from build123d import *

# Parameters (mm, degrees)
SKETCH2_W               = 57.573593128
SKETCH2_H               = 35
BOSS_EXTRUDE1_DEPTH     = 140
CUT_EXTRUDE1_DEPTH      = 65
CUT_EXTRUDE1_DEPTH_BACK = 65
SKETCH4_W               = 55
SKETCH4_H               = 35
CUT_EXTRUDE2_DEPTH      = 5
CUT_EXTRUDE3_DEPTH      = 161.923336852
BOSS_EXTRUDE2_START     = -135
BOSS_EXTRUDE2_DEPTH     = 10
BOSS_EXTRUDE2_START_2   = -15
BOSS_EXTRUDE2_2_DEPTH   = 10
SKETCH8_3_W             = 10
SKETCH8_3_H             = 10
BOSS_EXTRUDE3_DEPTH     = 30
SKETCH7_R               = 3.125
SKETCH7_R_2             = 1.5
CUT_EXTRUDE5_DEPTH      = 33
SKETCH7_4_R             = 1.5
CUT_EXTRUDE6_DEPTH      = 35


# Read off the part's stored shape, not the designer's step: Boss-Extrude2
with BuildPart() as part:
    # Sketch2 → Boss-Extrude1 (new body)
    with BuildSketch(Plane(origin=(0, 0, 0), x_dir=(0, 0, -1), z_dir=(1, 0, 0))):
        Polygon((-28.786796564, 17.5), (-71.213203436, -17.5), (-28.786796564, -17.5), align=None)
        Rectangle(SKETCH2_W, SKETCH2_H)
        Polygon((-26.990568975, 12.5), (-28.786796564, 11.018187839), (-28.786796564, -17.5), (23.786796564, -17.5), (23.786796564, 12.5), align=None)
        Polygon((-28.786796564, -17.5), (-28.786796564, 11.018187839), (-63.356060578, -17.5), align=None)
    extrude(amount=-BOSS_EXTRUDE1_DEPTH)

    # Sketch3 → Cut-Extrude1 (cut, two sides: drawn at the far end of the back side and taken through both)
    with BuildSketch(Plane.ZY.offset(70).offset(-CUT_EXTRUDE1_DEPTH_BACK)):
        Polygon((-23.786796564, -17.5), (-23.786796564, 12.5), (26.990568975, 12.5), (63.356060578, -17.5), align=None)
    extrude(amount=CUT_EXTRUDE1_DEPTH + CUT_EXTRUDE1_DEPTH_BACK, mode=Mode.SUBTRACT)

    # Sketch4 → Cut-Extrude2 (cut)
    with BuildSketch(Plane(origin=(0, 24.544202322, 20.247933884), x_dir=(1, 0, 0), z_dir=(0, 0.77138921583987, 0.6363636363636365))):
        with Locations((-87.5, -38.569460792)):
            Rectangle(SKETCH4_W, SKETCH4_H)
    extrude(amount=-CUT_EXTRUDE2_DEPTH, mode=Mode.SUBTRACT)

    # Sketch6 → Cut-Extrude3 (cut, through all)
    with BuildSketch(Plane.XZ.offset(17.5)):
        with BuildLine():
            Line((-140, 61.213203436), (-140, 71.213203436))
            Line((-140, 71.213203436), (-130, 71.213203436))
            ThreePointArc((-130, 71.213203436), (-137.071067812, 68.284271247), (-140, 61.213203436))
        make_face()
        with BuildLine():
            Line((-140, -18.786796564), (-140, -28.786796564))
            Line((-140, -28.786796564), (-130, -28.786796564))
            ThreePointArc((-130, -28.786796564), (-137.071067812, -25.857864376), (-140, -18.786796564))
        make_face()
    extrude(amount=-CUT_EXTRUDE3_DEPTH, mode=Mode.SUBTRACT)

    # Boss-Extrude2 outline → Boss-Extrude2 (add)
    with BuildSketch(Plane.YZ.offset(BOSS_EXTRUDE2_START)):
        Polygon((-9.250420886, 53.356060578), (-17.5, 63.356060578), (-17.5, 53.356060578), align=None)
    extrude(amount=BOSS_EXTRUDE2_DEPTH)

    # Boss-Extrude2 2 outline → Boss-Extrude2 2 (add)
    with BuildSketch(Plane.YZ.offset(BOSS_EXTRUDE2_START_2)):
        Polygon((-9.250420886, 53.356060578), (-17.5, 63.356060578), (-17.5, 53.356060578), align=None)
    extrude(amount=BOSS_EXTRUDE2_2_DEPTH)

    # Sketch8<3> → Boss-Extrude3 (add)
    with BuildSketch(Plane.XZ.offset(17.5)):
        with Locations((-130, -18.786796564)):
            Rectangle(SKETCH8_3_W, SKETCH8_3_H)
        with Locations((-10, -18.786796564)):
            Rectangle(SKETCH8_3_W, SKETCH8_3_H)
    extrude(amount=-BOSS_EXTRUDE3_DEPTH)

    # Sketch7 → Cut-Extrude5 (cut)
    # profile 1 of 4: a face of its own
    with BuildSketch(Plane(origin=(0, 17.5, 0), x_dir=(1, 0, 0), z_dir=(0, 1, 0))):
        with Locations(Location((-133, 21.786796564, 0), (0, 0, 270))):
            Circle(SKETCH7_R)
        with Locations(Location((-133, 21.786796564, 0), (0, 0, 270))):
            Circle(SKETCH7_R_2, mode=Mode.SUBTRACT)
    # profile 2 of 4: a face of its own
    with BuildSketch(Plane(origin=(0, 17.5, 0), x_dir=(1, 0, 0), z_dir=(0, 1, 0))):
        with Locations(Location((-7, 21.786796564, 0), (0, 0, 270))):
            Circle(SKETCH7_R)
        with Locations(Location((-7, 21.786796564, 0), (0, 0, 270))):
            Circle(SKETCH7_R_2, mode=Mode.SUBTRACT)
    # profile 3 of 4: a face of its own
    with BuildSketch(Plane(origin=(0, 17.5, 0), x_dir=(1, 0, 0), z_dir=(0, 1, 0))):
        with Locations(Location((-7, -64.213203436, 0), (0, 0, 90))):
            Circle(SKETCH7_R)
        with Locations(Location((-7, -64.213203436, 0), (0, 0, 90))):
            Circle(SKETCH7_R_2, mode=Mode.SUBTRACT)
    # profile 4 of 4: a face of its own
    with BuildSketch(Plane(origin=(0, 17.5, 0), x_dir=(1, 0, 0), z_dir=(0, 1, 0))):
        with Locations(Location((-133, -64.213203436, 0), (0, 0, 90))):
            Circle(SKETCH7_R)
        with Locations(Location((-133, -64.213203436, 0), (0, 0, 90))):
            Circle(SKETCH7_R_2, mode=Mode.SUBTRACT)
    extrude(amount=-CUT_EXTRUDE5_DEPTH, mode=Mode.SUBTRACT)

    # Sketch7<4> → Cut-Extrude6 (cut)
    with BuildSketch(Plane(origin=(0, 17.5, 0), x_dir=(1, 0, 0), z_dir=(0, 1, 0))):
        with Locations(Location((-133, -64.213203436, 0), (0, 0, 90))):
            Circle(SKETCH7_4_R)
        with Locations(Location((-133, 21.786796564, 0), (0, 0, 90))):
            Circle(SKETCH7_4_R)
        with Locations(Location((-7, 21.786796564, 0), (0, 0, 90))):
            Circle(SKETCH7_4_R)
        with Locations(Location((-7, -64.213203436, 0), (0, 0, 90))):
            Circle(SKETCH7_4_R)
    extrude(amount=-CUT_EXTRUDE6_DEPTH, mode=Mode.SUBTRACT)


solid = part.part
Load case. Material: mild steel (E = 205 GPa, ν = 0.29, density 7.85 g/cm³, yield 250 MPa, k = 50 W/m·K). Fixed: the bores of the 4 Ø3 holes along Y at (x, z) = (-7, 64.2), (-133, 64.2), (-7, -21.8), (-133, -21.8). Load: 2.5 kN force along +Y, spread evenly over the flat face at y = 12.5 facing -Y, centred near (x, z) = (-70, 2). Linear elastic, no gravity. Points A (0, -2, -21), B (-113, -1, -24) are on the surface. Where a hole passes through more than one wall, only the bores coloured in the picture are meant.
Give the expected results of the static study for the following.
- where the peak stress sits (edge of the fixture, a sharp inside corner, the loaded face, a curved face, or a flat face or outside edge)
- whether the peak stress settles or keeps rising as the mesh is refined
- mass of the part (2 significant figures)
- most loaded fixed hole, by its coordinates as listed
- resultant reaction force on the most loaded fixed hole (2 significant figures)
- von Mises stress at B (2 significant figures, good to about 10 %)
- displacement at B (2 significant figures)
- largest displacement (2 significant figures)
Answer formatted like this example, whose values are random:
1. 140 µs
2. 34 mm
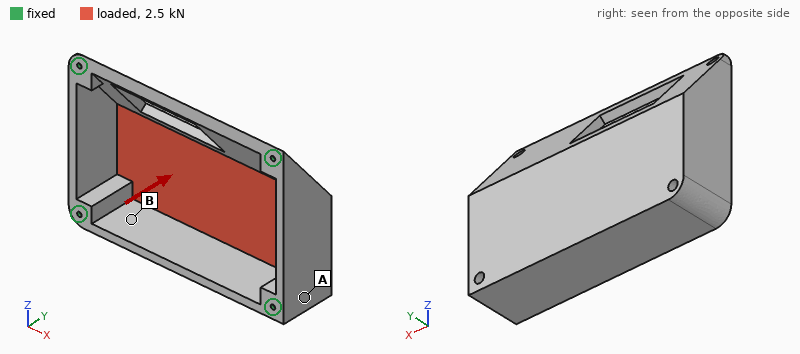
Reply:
1. edge of the fixture
2. keeps rising
3. 870 g
4. (-133, -21.8)
5. 1.2 kN
6. 15 MPa
7. 5.3 µm
8. 22 µm
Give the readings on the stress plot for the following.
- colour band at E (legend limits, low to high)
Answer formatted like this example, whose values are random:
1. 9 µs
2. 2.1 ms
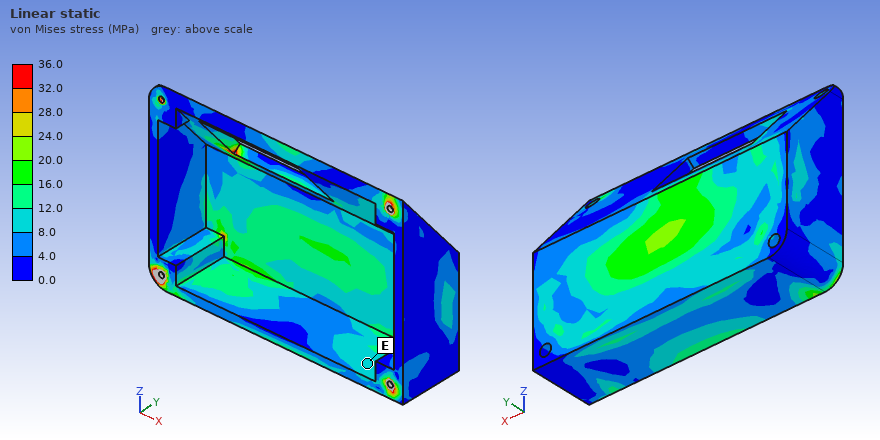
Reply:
1. 8.0 to 12.0 MPa
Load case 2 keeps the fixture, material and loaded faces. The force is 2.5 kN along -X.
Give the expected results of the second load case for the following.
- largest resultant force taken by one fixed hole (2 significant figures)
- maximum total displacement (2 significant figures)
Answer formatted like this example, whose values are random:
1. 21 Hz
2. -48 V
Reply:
1. 1.1 kN
2. 11 µm
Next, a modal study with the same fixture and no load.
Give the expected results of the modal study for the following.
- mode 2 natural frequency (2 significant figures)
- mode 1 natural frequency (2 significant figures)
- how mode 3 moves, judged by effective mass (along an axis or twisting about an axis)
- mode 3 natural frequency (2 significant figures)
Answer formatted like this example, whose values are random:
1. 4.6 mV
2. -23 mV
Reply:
1. 3000 Hz
2. 2100 Hz
3. along X
4. 3800 Hz
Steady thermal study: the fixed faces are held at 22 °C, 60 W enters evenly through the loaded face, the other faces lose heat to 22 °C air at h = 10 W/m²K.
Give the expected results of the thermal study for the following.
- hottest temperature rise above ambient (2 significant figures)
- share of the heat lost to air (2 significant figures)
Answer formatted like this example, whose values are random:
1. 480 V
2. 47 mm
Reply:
1. 76 K
2. 31 %
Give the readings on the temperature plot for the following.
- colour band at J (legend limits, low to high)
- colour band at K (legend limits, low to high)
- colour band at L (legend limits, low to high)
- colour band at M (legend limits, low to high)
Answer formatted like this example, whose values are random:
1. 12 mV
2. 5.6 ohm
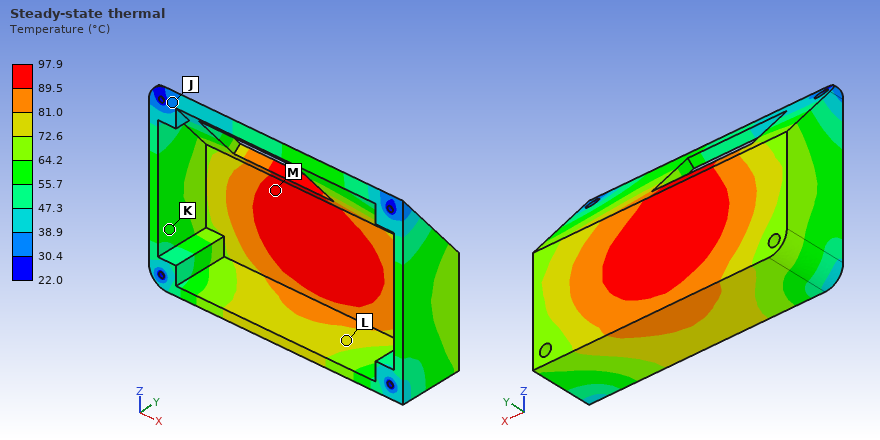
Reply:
1. 30.4 to 38.9 °C
2. 55.7 to 64.2 °C
3. 72.6 to 81.0 °C
4. 89.5 to 97.9 °C
